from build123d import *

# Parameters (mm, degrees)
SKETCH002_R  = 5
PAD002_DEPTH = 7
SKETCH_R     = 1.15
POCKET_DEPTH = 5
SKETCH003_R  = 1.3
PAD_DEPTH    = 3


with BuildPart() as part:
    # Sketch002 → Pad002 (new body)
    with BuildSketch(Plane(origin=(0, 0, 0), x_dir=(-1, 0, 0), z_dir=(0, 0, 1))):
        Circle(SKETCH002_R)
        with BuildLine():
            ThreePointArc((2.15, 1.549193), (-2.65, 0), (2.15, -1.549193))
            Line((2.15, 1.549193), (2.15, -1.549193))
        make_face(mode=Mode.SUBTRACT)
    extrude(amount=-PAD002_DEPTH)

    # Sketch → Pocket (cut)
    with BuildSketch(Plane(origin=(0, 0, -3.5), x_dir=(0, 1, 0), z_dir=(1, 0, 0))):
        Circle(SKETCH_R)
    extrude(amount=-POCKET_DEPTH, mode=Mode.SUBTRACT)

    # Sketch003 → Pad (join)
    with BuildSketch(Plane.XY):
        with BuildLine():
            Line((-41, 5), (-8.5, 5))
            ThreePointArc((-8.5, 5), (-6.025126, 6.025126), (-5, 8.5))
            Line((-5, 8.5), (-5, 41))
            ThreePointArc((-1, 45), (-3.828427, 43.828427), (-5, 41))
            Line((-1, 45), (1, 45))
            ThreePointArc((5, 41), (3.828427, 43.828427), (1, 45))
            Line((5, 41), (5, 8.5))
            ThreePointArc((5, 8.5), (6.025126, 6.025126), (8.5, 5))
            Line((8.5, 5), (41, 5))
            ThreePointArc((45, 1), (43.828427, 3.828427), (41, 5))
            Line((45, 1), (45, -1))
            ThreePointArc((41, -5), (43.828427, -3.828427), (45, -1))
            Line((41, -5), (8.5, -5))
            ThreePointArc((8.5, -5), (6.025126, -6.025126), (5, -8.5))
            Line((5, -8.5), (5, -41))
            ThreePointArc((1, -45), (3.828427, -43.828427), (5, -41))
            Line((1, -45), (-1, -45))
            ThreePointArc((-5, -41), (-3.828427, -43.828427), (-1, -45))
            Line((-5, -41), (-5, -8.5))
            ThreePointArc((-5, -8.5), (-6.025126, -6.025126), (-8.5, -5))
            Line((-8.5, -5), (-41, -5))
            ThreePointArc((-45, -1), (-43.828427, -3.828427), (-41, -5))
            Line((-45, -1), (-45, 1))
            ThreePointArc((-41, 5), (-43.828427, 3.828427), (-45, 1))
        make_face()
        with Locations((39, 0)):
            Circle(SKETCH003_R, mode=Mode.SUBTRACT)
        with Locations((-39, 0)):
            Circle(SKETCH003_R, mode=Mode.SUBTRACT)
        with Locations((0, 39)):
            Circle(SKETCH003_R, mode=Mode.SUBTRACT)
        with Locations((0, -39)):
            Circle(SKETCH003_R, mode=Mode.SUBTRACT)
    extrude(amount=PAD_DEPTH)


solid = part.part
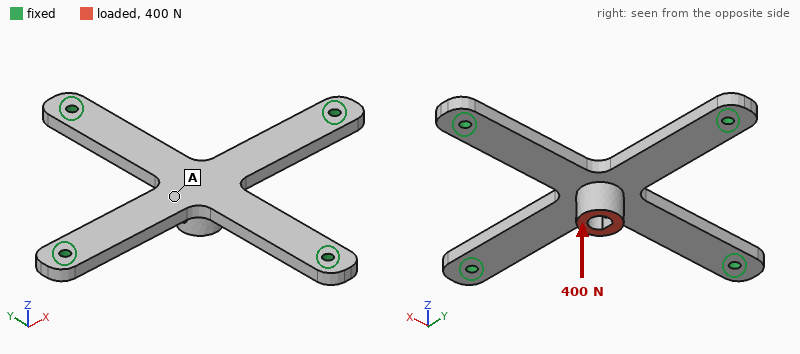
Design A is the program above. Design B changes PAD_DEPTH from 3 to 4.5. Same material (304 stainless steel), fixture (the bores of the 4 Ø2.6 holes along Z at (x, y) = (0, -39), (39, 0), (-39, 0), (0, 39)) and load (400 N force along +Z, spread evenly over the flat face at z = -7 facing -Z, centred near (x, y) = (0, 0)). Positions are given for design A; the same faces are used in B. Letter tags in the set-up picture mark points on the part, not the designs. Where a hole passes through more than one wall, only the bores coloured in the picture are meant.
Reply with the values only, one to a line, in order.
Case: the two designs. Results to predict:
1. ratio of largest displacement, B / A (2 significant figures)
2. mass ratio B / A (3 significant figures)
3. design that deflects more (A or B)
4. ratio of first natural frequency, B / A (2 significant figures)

0.32
1.46
A
1.5
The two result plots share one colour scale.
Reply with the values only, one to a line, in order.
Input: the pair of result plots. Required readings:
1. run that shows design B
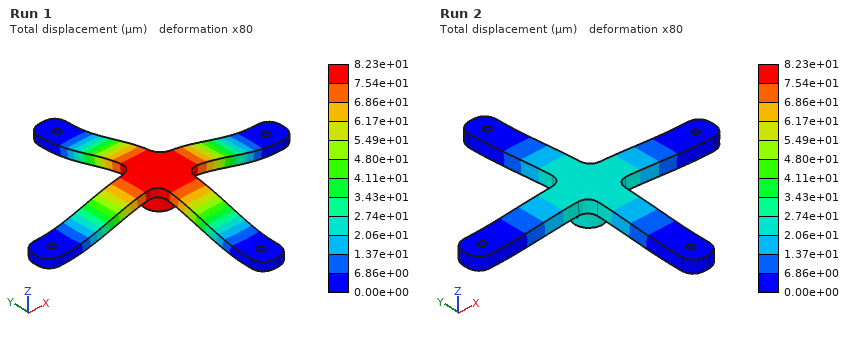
Run 2
